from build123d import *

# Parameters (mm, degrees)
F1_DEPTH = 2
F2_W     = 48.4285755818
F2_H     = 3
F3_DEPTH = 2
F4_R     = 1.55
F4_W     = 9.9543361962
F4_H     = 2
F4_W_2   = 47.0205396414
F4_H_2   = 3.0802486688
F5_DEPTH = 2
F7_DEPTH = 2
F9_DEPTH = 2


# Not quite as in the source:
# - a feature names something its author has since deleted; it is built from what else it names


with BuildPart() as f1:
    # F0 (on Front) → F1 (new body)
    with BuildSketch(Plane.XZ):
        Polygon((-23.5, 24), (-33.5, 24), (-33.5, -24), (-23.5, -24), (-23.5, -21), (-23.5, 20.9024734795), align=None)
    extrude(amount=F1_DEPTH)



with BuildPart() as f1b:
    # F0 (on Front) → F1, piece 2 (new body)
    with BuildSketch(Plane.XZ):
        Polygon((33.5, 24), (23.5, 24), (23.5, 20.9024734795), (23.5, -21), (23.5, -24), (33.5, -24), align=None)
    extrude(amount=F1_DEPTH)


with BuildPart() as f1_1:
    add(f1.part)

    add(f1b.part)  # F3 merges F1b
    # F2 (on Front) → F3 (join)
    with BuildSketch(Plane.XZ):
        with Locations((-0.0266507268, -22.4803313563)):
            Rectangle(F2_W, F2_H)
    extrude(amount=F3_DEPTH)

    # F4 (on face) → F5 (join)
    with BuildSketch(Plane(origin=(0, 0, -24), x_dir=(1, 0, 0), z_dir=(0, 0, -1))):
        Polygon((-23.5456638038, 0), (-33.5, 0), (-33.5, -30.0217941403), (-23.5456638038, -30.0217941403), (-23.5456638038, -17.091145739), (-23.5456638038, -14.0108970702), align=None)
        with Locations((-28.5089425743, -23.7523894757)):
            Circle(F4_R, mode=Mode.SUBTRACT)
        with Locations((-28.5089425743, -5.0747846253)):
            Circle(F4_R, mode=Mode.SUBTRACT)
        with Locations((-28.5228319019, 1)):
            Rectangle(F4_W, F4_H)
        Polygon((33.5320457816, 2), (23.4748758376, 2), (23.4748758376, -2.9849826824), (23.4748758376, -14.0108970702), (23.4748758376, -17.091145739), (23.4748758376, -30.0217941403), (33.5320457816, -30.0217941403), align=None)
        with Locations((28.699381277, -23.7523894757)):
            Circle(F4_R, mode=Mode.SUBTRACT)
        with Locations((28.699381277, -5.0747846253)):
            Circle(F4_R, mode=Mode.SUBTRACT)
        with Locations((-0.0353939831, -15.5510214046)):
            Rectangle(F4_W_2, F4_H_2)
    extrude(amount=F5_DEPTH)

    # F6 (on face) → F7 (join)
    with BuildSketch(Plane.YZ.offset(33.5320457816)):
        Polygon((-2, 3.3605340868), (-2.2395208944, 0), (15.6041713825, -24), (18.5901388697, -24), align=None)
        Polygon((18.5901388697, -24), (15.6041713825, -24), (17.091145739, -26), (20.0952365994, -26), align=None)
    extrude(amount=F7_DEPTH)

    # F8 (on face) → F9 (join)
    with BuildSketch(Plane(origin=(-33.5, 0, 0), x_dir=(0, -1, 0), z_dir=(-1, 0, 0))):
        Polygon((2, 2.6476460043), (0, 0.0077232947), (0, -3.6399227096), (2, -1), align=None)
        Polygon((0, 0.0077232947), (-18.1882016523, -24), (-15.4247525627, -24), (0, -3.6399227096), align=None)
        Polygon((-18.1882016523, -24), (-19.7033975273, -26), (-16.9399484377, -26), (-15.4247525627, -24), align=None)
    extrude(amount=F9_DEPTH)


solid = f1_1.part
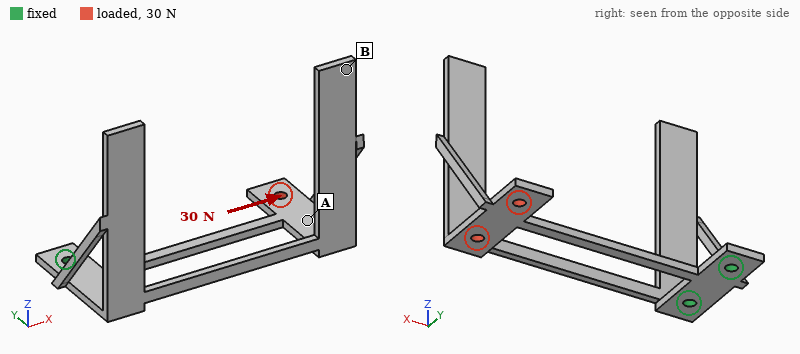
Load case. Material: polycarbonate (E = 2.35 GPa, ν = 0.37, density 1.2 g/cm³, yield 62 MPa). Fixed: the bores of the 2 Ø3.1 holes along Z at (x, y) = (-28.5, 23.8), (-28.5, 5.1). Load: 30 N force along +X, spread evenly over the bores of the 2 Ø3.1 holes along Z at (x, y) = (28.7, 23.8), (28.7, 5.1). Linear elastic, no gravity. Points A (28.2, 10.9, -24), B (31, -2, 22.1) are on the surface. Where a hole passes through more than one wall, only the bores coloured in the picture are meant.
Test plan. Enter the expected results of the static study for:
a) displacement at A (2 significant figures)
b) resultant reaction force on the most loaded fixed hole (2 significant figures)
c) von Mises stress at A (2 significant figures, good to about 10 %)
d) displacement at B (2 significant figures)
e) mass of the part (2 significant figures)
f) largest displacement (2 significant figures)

0.50 mm
16 N
1.5 MPa
0.95 mm
4.8 g
1.0 mm
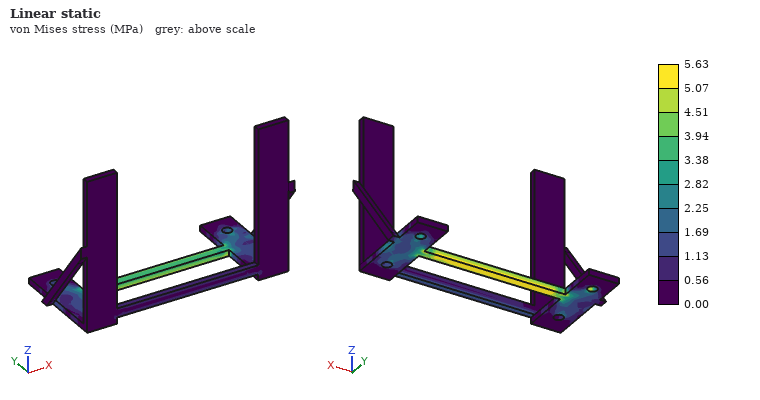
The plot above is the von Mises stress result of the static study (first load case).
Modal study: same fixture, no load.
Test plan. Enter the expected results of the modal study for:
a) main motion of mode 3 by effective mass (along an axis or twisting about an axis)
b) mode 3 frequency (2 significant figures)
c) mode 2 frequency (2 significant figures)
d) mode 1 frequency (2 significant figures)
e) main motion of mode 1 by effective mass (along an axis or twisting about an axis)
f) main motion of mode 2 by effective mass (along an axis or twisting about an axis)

along Y
170 Hz
64 Hz
49 Hz
along Z
along Y
